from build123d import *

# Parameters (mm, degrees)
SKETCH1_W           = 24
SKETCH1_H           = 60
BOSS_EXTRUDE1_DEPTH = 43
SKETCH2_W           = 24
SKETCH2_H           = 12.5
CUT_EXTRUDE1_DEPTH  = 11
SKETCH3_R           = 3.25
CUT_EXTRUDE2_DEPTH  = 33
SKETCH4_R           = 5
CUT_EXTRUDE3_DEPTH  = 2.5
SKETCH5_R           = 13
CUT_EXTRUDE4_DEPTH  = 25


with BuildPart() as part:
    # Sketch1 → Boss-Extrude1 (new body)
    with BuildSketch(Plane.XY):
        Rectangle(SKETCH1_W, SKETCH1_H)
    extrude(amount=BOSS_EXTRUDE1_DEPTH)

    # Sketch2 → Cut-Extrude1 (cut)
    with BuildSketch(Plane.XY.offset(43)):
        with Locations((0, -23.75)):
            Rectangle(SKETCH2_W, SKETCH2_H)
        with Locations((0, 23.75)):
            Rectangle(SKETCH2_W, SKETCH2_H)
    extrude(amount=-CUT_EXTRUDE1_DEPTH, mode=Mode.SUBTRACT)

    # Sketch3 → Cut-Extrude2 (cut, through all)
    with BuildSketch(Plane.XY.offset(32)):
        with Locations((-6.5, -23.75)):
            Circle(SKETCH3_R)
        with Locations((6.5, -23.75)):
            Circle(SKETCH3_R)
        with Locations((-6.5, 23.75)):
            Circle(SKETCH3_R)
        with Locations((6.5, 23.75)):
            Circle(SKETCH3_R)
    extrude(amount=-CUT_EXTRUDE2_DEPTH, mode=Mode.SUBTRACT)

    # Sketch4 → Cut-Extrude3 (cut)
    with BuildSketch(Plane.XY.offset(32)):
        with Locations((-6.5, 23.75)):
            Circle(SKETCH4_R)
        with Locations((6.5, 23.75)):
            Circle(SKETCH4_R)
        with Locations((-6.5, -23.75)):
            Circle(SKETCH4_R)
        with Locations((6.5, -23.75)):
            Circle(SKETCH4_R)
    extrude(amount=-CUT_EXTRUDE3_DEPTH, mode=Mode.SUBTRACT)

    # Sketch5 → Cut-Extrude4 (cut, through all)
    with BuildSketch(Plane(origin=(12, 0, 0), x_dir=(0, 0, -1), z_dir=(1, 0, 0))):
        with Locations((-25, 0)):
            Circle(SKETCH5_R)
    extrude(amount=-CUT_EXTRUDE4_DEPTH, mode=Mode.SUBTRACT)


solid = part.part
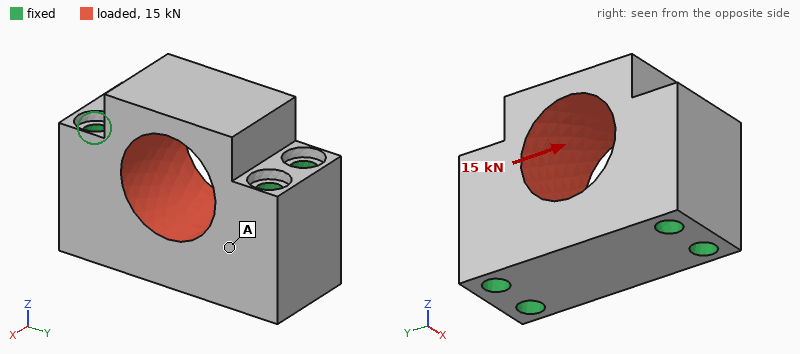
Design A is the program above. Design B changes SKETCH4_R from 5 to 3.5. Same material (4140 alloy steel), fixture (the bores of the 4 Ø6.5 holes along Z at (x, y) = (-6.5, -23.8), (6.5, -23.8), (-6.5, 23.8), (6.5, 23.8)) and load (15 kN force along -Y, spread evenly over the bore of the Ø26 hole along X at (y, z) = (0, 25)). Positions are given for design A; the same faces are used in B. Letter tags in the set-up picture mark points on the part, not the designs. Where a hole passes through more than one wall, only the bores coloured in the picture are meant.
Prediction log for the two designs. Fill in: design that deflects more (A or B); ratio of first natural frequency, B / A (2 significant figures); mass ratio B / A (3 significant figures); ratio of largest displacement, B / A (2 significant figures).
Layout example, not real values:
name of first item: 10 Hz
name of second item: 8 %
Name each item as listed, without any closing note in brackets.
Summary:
design that deflects more: A
ratio of first natural frequency, B / A: 1.0
mass ratio B / A: 1.01
ratio of largest displacement, B / A: 0.90
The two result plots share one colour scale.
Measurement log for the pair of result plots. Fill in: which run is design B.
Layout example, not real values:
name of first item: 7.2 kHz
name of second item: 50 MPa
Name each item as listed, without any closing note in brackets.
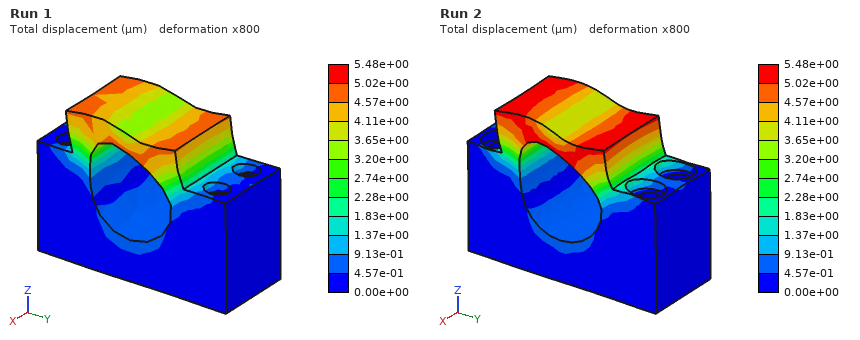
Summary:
which run is design B: Run 1
